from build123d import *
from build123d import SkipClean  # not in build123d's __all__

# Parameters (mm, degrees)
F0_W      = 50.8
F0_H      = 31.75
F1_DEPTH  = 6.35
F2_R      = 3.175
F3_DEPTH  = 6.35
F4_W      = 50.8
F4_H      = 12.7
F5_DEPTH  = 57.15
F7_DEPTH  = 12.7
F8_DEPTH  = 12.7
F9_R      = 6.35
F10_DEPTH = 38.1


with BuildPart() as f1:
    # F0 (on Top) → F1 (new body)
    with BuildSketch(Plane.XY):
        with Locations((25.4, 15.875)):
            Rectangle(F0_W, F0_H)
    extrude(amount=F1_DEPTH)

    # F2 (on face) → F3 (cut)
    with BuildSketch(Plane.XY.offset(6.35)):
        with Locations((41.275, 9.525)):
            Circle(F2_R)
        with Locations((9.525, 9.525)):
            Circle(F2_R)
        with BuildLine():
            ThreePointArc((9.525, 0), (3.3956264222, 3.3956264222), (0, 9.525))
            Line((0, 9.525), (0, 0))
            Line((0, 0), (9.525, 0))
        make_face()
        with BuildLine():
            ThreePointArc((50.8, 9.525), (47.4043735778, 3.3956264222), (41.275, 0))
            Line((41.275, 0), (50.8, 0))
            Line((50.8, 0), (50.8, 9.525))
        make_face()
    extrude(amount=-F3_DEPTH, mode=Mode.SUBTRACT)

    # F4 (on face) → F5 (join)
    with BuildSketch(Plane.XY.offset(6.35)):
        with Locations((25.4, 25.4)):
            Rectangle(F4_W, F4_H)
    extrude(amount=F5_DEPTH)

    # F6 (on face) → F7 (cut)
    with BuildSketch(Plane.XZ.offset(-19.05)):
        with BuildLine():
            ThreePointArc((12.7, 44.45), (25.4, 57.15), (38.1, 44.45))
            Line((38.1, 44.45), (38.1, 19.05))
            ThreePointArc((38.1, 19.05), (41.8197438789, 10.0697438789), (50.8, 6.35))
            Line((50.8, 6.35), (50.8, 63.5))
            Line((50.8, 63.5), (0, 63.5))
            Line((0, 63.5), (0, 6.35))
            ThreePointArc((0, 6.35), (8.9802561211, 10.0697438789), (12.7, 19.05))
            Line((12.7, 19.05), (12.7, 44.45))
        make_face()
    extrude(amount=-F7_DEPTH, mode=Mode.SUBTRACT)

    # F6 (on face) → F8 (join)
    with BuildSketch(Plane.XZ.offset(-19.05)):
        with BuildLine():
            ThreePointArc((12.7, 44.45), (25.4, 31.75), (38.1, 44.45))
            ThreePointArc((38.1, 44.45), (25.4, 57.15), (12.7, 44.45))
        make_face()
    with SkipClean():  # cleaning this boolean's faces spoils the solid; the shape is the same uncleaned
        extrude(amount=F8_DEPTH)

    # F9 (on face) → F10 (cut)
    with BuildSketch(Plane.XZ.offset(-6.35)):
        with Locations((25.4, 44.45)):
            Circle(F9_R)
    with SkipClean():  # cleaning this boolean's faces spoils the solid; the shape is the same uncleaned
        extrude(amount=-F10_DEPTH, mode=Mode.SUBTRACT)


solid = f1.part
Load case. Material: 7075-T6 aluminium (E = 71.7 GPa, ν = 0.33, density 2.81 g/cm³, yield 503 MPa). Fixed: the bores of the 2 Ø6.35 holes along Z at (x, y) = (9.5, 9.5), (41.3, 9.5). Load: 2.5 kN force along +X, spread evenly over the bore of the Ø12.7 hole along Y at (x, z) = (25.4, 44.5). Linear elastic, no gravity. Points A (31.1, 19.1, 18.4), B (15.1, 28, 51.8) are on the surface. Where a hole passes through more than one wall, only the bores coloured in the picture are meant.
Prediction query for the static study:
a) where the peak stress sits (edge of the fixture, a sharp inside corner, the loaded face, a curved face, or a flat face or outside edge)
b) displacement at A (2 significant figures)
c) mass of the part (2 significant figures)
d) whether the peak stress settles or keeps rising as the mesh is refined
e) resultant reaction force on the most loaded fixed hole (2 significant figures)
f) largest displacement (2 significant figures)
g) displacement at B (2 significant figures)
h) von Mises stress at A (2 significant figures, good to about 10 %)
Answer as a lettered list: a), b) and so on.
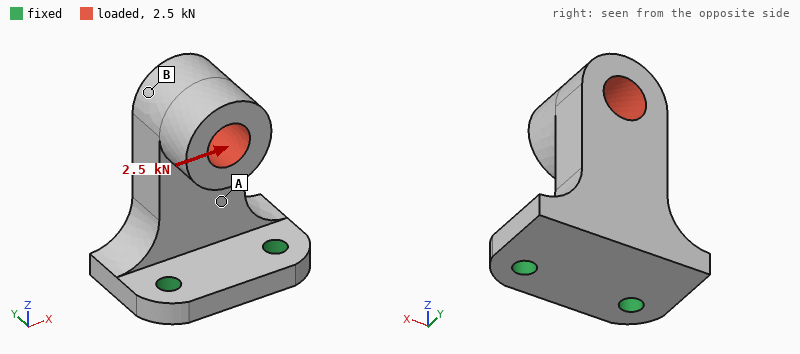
a) edge of the fixture
b) 0.052 mm
c) 82 g
d) keeps rising
e) 3.4 kN
f) 0.23 mm
g) 0.17 mm
h) 56 MPa
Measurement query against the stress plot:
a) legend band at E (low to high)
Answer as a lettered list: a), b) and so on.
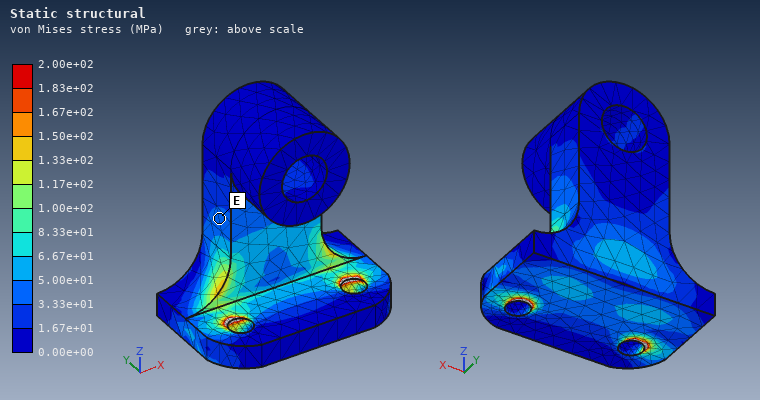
a) 3.33e+01 to 5.00e+01 MPa
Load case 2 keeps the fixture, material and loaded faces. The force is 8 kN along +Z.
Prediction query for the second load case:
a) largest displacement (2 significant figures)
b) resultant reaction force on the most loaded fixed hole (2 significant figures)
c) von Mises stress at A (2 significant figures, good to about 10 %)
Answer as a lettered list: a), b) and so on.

a) 0.13 mm
b) 4.0 kN
c) 86 MPa
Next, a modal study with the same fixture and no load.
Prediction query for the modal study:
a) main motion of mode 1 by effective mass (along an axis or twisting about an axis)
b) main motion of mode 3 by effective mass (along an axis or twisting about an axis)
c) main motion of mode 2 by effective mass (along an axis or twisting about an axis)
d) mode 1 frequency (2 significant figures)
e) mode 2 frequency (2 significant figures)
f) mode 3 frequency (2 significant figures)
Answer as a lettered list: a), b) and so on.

a) along Y
b) along Z
c) along X
d) 1500 Hz
e) 3400 Hz
f) 6500 Hz
